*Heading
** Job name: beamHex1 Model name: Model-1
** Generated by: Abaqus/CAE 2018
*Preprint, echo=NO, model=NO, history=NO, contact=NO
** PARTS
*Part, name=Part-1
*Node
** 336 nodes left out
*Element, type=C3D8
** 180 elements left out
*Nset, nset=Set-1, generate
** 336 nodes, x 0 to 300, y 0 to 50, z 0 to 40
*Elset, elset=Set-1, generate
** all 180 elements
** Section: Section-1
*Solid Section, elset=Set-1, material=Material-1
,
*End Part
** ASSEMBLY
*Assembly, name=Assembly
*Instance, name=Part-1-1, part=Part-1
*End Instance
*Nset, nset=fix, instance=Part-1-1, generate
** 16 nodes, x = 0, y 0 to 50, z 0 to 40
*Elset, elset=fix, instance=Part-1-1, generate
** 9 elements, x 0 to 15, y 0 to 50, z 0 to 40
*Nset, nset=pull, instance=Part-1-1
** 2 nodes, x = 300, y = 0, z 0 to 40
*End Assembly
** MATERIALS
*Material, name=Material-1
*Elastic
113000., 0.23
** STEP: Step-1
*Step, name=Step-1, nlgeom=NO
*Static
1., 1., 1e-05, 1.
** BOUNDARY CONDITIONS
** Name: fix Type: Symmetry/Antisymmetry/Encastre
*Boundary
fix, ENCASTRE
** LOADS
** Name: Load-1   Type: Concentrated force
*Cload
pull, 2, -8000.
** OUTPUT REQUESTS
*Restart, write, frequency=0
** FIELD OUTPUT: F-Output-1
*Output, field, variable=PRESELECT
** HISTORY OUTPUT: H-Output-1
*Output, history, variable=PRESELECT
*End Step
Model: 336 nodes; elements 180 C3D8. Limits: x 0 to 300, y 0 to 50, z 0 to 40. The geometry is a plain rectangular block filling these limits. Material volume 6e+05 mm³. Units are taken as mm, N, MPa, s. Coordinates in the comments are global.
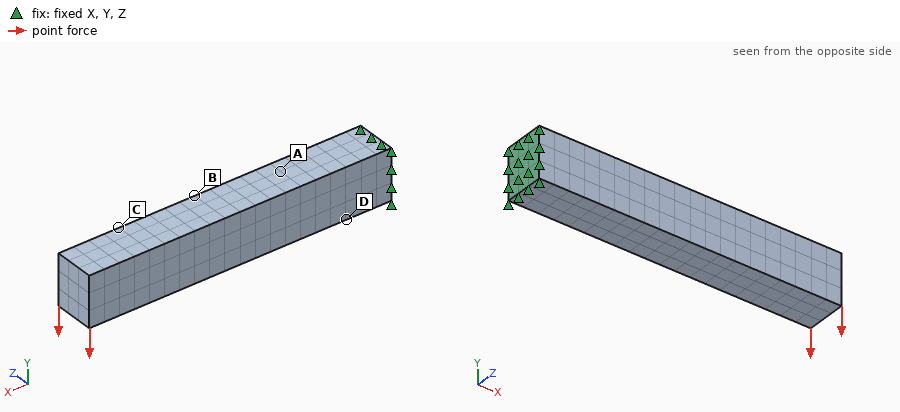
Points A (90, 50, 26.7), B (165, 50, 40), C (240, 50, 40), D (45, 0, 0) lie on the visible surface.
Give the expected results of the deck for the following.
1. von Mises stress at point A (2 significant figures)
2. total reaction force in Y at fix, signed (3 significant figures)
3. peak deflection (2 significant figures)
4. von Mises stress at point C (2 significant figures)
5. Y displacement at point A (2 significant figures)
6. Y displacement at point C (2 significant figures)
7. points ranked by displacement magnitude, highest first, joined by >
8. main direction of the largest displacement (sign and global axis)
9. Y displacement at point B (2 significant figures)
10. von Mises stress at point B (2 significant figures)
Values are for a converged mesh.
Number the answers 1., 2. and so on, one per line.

1. 200 MPa
2. 16000 N
3. 3.2 mm
4. 58 MPa
5. -0.39 mm
6. -2.2 mm
7. C > B > A > D
8. -Y
9. -1.2 mm
10. 130 MPa
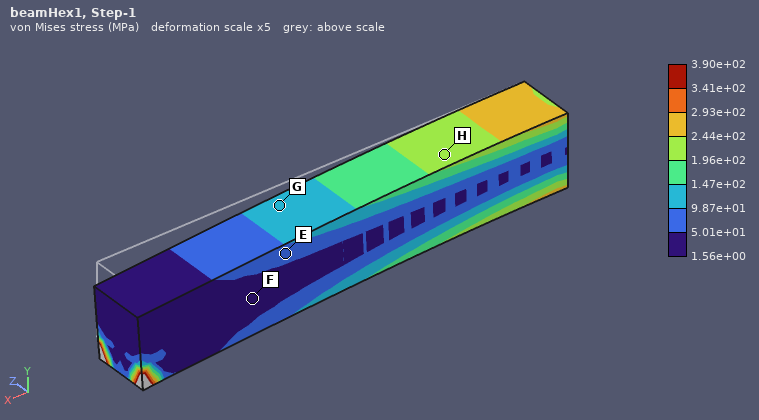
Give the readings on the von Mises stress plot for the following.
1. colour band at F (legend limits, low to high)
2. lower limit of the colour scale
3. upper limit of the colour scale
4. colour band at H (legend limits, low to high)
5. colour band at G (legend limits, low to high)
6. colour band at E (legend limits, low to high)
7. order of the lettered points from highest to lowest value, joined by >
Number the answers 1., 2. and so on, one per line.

1. 1.56e+00 to 5.01e+01 MPa
2. 1.56e+00 MPa
3. 3.90e+02 MPa
4. 1.96e+02 to 2.44e+02 MPa
5. 9.87e+01 to 1.47e+02 MPa
6. 5.01e+01 to 9.87e+01 MPa
7. H > G > E > F
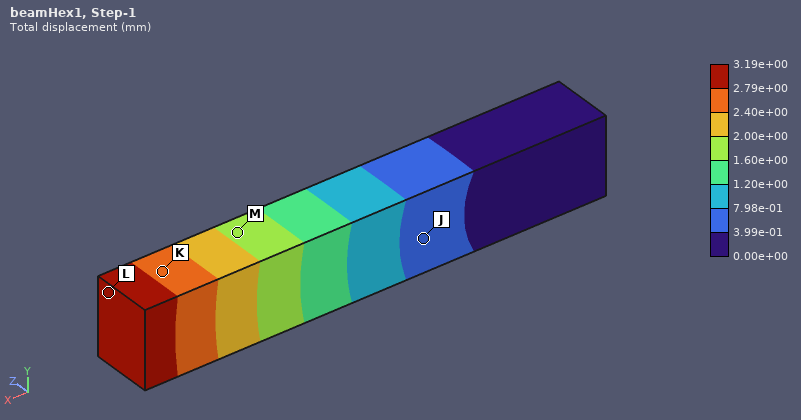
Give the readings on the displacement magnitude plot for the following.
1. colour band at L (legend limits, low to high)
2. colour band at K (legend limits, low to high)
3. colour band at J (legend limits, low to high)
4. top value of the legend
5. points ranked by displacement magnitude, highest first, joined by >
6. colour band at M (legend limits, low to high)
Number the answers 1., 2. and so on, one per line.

1. 2.79e+00 to 3.19e+00 mm
2. 2.40e+00 to 2.79e+00 mm
3. 3.99e-01 to 7.98e-01 mm
4. 3.19e+00 mm
5. L > K > M > J
6. 1.60e+00 to 2.00e+00 mm
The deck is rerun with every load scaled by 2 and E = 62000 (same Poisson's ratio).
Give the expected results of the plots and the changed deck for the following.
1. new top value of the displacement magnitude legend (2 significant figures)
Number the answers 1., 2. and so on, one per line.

1. 12 mm
